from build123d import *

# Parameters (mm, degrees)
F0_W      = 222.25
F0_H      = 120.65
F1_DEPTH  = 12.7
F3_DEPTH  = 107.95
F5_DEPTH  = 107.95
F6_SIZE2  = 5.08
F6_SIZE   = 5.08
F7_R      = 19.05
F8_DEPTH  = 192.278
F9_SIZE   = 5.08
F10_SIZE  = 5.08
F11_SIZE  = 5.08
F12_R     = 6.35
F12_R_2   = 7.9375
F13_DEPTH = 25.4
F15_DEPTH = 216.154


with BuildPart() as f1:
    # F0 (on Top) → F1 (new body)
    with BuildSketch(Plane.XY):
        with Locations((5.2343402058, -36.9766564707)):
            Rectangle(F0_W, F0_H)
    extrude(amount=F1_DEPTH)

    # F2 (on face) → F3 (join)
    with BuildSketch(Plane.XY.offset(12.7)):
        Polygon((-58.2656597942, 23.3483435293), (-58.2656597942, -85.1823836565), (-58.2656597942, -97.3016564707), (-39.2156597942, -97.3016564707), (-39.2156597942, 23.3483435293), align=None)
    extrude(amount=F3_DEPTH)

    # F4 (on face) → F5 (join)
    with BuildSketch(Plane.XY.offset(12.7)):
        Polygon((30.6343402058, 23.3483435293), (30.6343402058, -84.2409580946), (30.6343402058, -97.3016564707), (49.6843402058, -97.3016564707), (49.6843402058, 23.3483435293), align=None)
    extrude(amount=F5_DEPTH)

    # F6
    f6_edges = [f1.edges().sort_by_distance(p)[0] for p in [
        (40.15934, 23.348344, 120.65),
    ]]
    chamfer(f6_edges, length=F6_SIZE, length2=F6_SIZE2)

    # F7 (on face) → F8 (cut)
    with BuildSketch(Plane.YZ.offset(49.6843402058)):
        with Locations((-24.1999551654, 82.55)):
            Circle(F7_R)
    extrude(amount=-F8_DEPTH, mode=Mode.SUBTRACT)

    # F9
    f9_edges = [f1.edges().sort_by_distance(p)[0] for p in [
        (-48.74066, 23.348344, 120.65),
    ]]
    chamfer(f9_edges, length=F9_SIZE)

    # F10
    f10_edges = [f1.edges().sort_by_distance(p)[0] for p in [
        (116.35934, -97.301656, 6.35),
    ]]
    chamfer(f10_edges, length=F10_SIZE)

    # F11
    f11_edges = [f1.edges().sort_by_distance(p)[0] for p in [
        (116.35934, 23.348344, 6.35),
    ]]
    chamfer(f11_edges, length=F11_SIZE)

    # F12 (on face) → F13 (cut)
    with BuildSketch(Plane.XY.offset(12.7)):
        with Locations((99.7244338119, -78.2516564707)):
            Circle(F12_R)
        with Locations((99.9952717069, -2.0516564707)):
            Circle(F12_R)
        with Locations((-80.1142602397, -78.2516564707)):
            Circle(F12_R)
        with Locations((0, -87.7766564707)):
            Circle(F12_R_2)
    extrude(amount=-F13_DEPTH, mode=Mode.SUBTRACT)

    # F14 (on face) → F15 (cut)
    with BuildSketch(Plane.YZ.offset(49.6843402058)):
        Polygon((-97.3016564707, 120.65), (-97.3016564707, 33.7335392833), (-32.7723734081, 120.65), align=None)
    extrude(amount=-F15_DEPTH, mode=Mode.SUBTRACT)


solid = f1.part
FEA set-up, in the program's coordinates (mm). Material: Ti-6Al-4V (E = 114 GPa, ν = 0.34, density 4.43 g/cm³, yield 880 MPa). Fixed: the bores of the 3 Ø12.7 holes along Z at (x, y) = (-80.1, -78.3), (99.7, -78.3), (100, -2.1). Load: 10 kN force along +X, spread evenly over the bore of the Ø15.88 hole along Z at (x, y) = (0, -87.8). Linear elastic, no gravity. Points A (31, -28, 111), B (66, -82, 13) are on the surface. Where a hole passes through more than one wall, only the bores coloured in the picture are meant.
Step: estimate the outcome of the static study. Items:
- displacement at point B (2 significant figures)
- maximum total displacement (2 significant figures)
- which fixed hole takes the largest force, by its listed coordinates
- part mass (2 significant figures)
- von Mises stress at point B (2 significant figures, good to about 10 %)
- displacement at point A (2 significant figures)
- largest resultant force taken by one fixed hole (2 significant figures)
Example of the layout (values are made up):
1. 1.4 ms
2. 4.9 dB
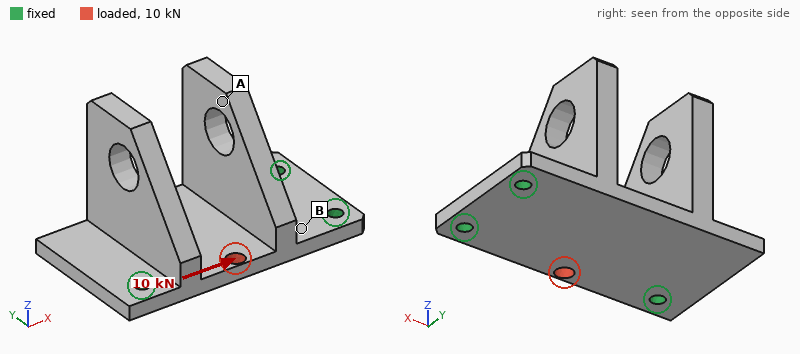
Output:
1. 2.5 µm
2. 11 µm
3. (-80.1, -78.3)
4. 3.0 kg
5. 8.4 MPa
6. 2.6 µm
7. 4.8 kN
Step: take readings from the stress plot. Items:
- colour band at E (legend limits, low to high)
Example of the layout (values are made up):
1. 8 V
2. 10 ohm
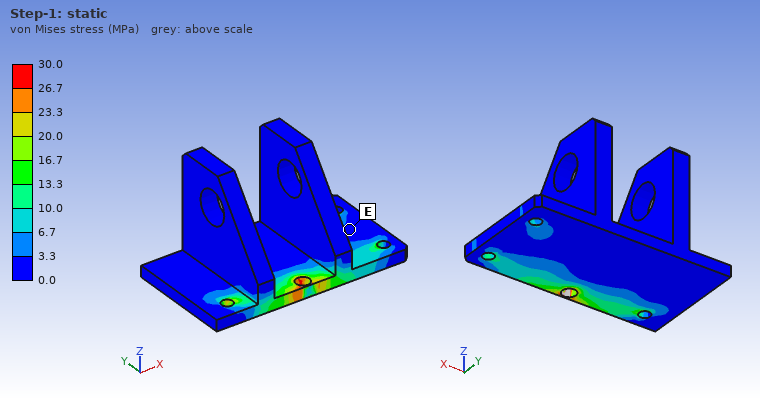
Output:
1. 0.0 to 3.3 MPa
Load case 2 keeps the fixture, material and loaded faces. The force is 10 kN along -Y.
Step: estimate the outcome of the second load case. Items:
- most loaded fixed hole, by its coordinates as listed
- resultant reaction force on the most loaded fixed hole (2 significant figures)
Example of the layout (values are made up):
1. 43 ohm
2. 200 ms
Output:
1. (-80.1, -78.3)
2. 5.0 kN
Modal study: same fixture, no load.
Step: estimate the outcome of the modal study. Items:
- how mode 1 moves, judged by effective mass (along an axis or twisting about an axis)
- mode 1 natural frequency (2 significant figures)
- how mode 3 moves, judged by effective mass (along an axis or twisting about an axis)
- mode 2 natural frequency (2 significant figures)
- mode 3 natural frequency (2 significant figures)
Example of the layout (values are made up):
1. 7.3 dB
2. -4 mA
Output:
1. along Z
2. 640 Hz
3. along X
4. 820 Hz
5. 1300 Hz
